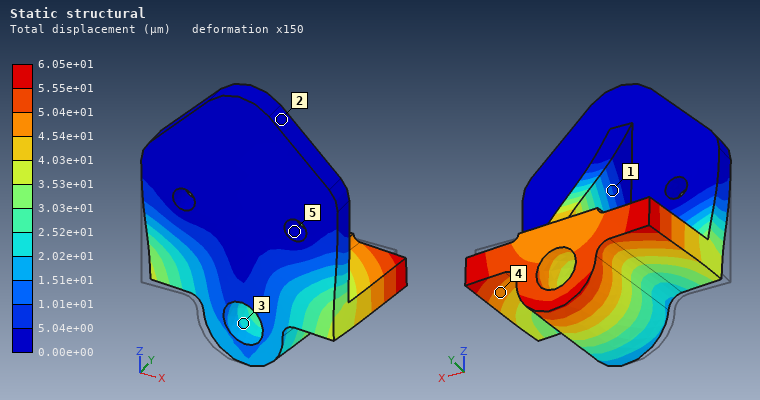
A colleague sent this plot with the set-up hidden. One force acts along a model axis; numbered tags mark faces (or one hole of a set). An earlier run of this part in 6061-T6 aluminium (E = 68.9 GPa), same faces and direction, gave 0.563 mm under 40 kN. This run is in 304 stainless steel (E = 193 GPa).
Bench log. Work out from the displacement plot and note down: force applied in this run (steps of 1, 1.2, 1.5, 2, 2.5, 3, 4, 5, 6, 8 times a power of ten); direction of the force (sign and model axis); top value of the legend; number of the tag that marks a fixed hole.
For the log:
12 kN
+X
6.05e+01 µm
5
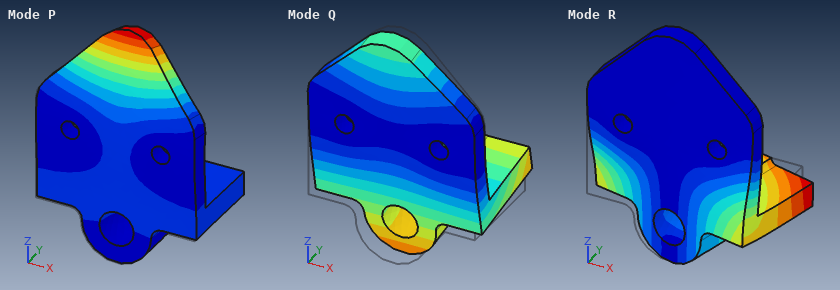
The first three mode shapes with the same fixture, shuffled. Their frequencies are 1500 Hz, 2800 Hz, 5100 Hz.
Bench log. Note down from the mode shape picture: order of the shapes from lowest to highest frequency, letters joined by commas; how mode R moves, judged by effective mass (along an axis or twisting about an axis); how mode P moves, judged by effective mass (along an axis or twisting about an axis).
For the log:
Q, R, P
along X
along Y
